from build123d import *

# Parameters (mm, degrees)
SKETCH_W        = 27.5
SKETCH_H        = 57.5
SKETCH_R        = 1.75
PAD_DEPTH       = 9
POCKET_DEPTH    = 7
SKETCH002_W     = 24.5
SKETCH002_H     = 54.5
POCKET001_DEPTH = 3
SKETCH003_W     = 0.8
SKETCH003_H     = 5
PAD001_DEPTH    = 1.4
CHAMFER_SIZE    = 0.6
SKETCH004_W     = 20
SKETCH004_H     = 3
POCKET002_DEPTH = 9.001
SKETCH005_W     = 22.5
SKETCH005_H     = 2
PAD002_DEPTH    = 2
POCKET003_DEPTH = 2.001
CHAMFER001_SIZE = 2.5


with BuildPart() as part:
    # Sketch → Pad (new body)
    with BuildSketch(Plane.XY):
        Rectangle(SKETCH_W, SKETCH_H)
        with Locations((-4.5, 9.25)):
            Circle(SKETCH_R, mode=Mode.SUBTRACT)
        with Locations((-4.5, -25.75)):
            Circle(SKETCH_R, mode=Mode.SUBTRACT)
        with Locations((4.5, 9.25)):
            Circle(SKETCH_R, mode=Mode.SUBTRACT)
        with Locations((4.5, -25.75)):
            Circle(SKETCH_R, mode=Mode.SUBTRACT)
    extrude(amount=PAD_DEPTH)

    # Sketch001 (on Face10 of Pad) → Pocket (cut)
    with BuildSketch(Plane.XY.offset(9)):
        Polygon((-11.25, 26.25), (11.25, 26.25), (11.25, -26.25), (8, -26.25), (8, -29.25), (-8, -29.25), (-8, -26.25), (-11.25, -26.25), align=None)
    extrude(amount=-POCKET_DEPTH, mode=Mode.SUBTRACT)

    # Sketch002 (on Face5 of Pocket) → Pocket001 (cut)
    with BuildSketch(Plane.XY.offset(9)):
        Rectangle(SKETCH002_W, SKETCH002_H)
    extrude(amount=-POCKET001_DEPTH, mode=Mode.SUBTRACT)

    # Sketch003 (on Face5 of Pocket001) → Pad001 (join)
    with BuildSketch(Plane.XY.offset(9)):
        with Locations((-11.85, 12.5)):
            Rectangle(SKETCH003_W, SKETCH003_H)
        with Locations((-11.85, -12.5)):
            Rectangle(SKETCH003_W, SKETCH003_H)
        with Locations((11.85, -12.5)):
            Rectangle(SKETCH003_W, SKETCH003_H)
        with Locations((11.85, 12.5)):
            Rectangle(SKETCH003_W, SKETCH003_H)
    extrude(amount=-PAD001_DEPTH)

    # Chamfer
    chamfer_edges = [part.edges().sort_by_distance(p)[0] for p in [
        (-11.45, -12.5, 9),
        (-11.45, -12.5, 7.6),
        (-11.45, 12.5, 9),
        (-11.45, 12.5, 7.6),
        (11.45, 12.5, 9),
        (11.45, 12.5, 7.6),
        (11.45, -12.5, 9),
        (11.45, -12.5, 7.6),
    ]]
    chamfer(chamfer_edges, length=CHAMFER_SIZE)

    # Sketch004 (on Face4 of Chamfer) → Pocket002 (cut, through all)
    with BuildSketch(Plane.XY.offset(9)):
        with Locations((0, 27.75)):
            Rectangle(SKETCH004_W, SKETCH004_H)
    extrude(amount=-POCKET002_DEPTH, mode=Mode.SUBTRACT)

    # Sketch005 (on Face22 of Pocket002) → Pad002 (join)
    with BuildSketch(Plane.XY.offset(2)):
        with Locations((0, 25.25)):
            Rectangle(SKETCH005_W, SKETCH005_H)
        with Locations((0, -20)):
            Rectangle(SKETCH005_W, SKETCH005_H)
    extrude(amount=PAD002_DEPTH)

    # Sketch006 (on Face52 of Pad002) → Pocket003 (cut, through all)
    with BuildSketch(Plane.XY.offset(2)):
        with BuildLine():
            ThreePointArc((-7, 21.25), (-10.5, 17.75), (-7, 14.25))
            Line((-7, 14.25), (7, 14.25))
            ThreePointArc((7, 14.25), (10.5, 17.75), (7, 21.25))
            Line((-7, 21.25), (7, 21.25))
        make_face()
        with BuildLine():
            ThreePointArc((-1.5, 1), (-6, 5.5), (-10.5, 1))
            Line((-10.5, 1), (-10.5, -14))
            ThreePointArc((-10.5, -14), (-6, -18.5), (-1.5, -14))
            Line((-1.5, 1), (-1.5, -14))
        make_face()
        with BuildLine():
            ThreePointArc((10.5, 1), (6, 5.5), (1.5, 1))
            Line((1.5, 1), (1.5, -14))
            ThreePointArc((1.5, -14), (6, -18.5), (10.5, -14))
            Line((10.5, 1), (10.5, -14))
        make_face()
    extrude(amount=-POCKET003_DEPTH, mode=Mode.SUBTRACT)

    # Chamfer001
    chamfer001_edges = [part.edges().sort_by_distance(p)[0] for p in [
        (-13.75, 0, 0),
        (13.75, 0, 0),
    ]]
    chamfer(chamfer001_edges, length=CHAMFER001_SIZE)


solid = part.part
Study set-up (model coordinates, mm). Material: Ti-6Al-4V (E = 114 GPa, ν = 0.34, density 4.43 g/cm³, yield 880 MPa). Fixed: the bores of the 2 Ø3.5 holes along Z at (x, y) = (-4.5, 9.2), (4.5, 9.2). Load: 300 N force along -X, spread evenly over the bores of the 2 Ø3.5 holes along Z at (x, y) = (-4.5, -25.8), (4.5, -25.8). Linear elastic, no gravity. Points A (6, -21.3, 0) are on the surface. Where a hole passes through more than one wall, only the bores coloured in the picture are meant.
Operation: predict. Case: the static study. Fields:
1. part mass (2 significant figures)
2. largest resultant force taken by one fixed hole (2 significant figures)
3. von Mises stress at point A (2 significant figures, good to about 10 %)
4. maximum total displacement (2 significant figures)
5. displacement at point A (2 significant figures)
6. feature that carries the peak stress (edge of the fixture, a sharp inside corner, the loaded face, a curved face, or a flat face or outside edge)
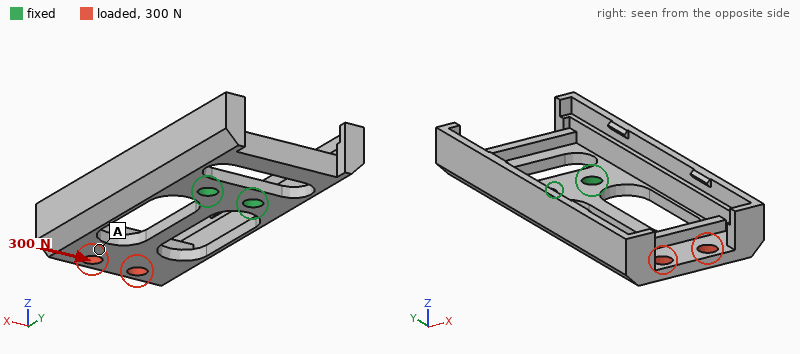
16 g
710 N
34 MPa
0.22 mm
0.18 mm
a curved face
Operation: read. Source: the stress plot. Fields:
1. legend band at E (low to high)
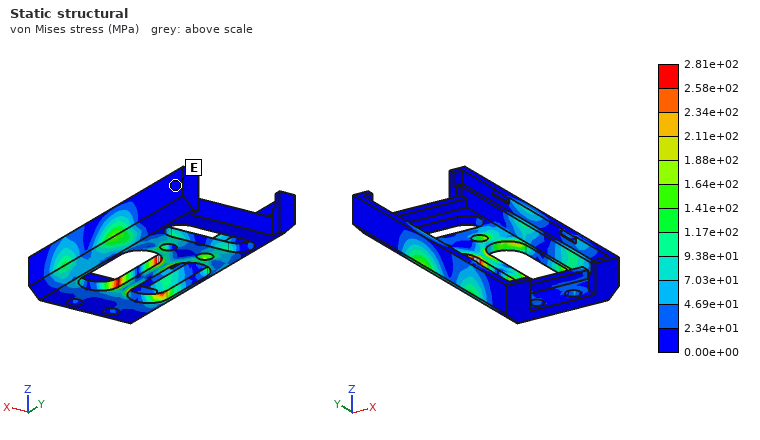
0.00e+00 to 2.34e+01 MPa
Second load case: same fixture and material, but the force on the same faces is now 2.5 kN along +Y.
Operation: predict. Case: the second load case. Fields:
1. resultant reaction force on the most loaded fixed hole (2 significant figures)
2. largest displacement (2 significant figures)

1.3 kN
0.11 mm
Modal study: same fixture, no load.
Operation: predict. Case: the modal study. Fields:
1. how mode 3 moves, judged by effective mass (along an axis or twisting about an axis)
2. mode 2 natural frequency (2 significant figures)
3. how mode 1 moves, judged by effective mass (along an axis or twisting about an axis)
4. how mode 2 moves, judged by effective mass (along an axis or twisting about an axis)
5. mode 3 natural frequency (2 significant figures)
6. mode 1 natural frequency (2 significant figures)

along X
2200 Hz
along Z
along X
2900 Hz
1300 Hz
